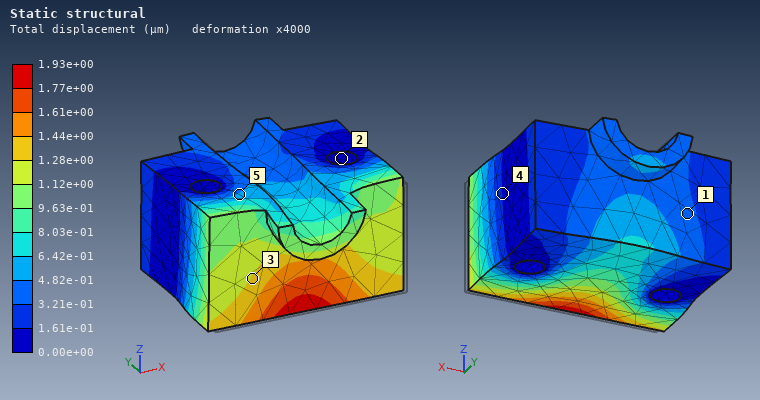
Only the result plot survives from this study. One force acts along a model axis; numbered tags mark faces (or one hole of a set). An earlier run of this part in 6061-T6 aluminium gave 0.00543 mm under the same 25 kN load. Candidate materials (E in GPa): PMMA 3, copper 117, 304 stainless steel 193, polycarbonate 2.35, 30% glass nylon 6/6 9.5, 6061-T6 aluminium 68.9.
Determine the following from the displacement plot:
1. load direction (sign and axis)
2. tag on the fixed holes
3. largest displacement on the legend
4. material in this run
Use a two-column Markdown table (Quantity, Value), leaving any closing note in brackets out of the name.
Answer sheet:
| Quantity | Value |
|---|---|
| load direction | +Y |
| tag on the fixed holes | 2 |
| largest displacement on the legend | 1.93e+00 µm |
| material in this run | 304 stainless steel |
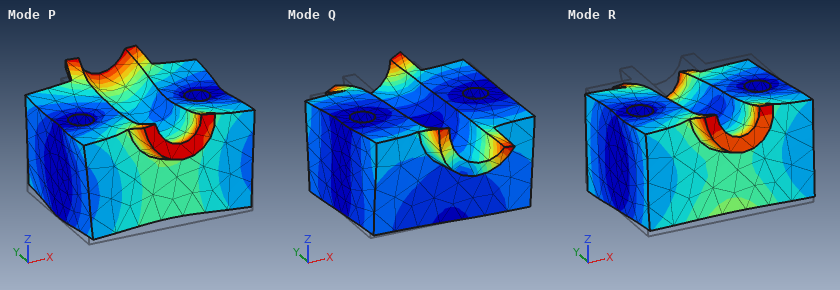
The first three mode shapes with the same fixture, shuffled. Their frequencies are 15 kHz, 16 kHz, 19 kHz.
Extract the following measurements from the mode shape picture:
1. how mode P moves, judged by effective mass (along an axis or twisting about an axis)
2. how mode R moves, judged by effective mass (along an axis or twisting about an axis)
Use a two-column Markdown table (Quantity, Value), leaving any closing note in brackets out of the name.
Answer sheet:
| Quantity | Value |
|---|---|
| how mode P moves, judged by effective mass | along Z |
| how mode R moves, judged by effective mass | twisting about X |
